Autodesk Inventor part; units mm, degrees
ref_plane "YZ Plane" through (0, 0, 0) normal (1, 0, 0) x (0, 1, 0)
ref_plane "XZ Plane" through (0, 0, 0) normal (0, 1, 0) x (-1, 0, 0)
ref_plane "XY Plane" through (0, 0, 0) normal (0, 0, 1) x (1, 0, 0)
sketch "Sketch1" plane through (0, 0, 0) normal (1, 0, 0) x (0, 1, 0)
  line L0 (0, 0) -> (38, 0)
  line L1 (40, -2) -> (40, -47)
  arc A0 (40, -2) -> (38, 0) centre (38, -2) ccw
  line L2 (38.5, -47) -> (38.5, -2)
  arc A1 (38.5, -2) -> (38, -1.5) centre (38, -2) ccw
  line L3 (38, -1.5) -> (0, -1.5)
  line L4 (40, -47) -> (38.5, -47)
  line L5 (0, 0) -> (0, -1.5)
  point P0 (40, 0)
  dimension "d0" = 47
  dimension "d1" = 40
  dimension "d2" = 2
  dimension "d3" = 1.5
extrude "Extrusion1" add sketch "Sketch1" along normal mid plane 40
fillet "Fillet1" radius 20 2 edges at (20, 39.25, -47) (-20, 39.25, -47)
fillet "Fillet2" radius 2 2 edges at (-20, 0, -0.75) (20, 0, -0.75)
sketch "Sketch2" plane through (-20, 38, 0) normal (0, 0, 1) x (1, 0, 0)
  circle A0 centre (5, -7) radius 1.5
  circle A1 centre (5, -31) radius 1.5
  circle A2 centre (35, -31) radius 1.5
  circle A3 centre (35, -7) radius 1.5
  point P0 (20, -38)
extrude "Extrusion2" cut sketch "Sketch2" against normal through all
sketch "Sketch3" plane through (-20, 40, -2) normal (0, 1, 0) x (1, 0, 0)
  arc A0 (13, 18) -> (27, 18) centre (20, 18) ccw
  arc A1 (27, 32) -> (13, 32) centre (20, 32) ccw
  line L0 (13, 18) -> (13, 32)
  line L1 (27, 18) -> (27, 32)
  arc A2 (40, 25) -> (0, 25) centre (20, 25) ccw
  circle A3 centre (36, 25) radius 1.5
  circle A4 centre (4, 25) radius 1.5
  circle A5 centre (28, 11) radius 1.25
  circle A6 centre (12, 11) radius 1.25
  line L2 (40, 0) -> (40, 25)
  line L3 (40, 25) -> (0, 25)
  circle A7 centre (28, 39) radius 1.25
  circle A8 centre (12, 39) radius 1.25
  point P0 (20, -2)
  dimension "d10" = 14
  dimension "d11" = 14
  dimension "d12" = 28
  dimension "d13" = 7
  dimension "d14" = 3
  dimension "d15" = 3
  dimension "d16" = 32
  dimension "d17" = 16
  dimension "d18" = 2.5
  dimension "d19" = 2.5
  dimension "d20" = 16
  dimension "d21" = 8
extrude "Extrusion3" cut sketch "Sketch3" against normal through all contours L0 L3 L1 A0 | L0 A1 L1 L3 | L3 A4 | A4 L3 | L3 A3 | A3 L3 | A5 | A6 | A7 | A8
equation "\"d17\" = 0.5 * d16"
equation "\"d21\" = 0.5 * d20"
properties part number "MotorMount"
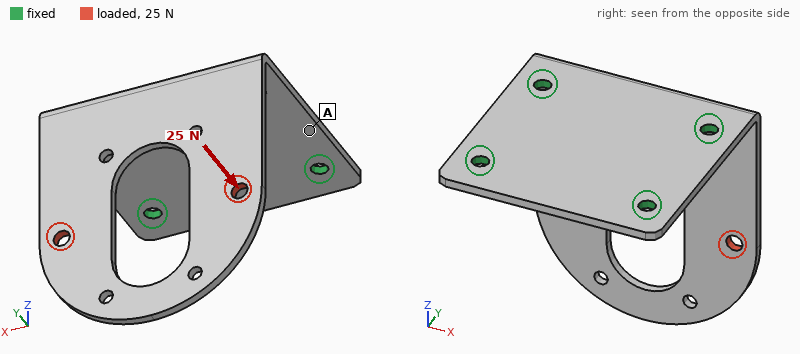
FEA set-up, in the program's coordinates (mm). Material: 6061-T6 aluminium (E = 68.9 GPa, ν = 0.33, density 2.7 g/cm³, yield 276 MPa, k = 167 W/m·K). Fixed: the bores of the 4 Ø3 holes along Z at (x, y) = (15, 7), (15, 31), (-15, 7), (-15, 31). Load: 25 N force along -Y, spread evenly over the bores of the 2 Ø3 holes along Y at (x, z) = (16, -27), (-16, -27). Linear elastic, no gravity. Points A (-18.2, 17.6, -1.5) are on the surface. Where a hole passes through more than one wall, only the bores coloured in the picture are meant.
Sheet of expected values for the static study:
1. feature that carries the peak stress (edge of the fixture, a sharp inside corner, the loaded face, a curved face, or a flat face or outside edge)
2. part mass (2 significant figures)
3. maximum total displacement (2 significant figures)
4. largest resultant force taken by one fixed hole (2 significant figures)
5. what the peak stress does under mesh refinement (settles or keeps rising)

edge of the fixture
11 g
0.75 mm
9.4 N
keeps rising
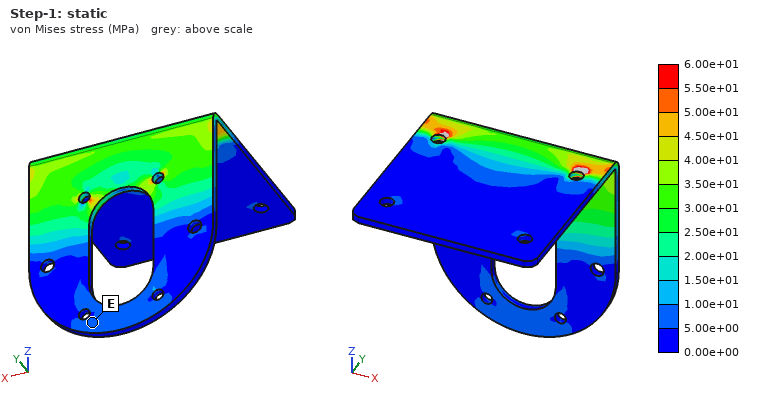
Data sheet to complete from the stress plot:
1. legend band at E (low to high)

5.00e+00 to 1.00e+01 MPa
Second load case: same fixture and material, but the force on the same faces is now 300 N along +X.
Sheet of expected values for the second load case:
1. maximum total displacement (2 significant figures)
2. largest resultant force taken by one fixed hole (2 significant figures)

0.37 mm
310 N
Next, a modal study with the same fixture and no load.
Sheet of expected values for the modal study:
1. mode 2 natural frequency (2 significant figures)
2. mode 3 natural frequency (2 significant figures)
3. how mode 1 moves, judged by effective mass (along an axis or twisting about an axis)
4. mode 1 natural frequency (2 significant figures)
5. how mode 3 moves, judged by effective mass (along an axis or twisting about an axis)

1600 Hz
2900 Hz
along Y
580 Hz
along X
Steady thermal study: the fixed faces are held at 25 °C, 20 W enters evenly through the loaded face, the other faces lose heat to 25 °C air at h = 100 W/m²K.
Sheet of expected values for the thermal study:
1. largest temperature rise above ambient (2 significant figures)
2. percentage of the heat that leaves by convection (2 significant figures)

61 K
53 %
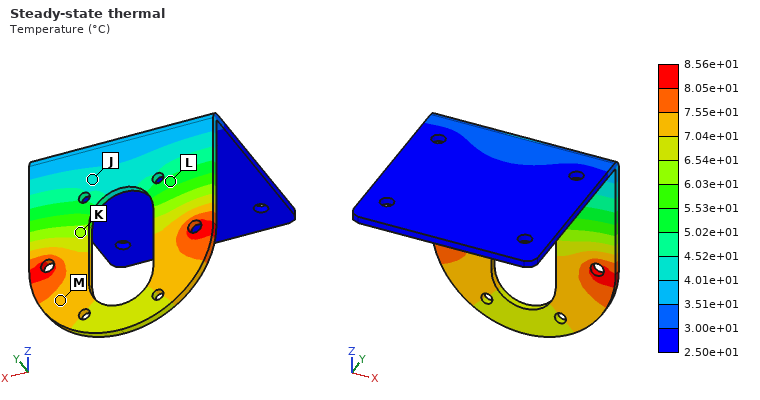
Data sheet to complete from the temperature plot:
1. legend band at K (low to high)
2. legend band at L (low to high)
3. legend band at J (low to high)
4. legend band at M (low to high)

6.03e+01 to 6.54e+01 °C
5.02e+01 to 5.53e+01 °C
4.01e+01 to 4.52e+01 °C
7.04e+01 to 7.55e+01 °C
